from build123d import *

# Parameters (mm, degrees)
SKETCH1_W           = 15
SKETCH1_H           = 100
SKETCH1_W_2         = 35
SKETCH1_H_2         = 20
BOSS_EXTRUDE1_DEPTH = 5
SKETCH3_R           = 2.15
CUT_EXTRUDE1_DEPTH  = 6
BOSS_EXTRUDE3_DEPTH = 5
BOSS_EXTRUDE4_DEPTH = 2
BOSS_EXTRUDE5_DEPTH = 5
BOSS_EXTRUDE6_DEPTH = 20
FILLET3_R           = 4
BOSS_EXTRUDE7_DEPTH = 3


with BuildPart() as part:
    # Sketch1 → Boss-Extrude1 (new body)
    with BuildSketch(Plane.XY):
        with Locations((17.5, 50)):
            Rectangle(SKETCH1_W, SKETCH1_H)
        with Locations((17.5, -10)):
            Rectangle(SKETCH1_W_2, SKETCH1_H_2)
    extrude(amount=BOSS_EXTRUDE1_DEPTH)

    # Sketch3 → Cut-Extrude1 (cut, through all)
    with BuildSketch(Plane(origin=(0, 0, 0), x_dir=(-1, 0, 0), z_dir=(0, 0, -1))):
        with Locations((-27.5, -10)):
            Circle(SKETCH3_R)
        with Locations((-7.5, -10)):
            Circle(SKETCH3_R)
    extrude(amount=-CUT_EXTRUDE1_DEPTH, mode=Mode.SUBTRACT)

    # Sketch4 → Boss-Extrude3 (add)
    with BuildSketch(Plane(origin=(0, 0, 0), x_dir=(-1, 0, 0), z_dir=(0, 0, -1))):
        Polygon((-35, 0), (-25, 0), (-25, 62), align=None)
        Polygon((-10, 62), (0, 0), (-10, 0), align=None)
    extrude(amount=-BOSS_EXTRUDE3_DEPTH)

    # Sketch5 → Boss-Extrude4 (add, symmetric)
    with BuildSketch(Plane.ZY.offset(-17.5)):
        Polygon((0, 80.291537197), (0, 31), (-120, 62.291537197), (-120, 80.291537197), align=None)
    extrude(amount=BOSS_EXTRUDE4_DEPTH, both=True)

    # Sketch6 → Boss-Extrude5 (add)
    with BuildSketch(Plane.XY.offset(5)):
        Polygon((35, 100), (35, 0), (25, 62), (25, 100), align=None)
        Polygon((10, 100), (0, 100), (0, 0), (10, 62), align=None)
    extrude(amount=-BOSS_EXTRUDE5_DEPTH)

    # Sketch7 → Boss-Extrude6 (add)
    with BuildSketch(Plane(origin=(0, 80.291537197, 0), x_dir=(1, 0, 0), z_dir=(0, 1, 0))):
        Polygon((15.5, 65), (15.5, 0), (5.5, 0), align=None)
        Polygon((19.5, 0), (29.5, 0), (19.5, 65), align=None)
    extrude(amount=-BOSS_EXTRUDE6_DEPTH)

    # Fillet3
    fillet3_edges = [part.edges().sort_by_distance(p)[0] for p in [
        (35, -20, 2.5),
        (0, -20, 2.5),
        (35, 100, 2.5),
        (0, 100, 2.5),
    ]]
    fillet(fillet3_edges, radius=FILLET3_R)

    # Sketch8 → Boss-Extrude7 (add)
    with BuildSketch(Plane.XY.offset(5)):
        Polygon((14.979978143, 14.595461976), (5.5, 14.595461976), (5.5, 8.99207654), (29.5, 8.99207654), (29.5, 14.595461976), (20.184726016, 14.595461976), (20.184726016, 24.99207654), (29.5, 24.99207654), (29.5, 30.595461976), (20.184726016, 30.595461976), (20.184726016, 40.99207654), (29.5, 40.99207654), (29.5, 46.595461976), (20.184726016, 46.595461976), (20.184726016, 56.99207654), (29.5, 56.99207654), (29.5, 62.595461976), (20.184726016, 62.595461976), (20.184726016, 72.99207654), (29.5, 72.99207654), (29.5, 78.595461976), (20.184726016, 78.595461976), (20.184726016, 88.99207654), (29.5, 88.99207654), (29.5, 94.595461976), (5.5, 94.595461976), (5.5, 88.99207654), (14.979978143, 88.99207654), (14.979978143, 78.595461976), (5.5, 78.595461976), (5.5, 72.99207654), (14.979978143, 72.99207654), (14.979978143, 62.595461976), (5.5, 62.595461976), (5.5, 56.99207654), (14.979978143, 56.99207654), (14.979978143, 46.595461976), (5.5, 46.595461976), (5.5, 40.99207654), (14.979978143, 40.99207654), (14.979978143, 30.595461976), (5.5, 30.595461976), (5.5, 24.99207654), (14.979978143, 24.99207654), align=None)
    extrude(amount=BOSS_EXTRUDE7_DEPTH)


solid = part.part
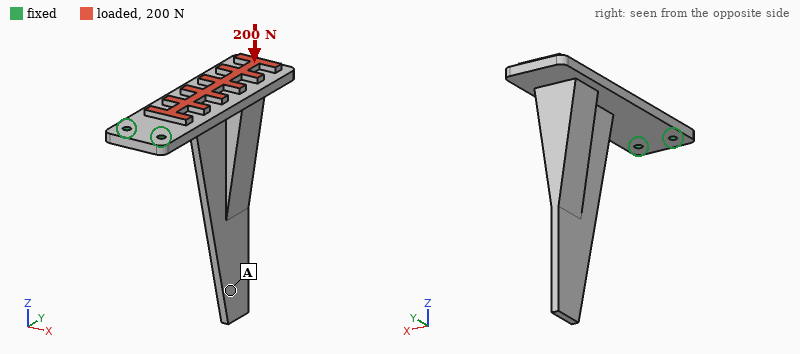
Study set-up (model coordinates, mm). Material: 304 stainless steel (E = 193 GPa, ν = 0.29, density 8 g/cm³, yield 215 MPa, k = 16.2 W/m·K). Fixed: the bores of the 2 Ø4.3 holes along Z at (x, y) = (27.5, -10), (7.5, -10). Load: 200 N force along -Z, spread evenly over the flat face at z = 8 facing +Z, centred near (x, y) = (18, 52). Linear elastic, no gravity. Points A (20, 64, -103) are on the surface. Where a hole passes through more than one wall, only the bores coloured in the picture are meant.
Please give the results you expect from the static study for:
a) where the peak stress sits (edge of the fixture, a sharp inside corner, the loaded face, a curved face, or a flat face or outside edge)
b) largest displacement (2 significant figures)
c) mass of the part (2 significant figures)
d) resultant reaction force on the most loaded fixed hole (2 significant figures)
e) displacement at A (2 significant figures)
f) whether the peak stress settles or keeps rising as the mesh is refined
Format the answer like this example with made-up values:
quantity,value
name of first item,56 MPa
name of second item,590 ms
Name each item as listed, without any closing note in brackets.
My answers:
quantity,value
where the peak stress sits,edge of the fixture
largest displacement,0.61 mm
mass of the part,430 g
resultant reaction force on the most loaded fixed hole,100 N
displacement at A,0.51 mm
whether the peak stress settles or keeps rising as the mesh is refined,keeps rising
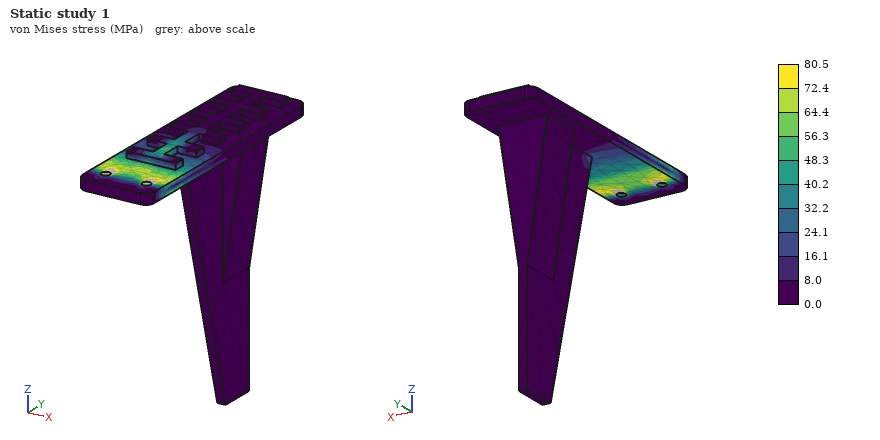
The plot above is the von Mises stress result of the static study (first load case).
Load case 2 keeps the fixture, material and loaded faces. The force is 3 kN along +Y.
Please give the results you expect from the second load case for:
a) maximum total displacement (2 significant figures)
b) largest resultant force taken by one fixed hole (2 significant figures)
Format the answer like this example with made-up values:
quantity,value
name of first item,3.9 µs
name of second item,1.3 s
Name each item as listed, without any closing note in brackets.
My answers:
quantity,value
maximum total displacement,1.1 mm
largest resultant force taken by one fixed hole,1.5 kN
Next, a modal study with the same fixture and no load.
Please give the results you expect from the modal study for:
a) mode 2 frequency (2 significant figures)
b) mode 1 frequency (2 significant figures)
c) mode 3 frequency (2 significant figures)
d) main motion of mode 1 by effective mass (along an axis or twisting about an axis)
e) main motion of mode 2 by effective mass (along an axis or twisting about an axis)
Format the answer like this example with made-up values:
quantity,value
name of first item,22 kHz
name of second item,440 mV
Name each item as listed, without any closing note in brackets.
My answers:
quantity,value
mode 2 frequency,310 Hz
mode 1 frequency,170 Hz
mode 3 frequency,1200 Hz
main motion of mode 1 by effective mass,along Z
main motion of mode 2 by effective mass,along X
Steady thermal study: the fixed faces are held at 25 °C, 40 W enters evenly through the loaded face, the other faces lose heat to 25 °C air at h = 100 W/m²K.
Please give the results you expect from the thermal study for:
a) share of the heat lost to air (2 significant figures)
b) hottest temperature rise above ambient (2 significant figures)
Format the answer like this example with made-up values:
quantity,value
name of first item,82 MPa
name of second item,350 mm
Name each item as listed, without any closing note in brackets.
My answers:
quantity,value
share of the heat lost to air,92 %
hottest temperature rise above ambient,51 K
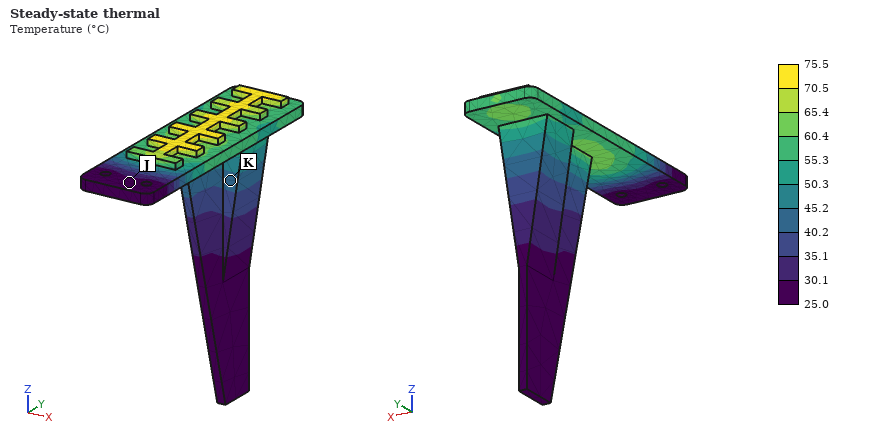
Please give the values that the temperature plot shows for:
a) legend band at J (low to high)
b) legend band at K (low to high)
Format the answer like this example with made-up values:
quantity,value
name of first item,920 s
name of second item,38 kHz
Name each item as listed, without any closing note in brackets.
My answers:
quantity,value
legend band at J,25.0 to 30.1 °C
legend band at K,40.2 to 45.2 °C
